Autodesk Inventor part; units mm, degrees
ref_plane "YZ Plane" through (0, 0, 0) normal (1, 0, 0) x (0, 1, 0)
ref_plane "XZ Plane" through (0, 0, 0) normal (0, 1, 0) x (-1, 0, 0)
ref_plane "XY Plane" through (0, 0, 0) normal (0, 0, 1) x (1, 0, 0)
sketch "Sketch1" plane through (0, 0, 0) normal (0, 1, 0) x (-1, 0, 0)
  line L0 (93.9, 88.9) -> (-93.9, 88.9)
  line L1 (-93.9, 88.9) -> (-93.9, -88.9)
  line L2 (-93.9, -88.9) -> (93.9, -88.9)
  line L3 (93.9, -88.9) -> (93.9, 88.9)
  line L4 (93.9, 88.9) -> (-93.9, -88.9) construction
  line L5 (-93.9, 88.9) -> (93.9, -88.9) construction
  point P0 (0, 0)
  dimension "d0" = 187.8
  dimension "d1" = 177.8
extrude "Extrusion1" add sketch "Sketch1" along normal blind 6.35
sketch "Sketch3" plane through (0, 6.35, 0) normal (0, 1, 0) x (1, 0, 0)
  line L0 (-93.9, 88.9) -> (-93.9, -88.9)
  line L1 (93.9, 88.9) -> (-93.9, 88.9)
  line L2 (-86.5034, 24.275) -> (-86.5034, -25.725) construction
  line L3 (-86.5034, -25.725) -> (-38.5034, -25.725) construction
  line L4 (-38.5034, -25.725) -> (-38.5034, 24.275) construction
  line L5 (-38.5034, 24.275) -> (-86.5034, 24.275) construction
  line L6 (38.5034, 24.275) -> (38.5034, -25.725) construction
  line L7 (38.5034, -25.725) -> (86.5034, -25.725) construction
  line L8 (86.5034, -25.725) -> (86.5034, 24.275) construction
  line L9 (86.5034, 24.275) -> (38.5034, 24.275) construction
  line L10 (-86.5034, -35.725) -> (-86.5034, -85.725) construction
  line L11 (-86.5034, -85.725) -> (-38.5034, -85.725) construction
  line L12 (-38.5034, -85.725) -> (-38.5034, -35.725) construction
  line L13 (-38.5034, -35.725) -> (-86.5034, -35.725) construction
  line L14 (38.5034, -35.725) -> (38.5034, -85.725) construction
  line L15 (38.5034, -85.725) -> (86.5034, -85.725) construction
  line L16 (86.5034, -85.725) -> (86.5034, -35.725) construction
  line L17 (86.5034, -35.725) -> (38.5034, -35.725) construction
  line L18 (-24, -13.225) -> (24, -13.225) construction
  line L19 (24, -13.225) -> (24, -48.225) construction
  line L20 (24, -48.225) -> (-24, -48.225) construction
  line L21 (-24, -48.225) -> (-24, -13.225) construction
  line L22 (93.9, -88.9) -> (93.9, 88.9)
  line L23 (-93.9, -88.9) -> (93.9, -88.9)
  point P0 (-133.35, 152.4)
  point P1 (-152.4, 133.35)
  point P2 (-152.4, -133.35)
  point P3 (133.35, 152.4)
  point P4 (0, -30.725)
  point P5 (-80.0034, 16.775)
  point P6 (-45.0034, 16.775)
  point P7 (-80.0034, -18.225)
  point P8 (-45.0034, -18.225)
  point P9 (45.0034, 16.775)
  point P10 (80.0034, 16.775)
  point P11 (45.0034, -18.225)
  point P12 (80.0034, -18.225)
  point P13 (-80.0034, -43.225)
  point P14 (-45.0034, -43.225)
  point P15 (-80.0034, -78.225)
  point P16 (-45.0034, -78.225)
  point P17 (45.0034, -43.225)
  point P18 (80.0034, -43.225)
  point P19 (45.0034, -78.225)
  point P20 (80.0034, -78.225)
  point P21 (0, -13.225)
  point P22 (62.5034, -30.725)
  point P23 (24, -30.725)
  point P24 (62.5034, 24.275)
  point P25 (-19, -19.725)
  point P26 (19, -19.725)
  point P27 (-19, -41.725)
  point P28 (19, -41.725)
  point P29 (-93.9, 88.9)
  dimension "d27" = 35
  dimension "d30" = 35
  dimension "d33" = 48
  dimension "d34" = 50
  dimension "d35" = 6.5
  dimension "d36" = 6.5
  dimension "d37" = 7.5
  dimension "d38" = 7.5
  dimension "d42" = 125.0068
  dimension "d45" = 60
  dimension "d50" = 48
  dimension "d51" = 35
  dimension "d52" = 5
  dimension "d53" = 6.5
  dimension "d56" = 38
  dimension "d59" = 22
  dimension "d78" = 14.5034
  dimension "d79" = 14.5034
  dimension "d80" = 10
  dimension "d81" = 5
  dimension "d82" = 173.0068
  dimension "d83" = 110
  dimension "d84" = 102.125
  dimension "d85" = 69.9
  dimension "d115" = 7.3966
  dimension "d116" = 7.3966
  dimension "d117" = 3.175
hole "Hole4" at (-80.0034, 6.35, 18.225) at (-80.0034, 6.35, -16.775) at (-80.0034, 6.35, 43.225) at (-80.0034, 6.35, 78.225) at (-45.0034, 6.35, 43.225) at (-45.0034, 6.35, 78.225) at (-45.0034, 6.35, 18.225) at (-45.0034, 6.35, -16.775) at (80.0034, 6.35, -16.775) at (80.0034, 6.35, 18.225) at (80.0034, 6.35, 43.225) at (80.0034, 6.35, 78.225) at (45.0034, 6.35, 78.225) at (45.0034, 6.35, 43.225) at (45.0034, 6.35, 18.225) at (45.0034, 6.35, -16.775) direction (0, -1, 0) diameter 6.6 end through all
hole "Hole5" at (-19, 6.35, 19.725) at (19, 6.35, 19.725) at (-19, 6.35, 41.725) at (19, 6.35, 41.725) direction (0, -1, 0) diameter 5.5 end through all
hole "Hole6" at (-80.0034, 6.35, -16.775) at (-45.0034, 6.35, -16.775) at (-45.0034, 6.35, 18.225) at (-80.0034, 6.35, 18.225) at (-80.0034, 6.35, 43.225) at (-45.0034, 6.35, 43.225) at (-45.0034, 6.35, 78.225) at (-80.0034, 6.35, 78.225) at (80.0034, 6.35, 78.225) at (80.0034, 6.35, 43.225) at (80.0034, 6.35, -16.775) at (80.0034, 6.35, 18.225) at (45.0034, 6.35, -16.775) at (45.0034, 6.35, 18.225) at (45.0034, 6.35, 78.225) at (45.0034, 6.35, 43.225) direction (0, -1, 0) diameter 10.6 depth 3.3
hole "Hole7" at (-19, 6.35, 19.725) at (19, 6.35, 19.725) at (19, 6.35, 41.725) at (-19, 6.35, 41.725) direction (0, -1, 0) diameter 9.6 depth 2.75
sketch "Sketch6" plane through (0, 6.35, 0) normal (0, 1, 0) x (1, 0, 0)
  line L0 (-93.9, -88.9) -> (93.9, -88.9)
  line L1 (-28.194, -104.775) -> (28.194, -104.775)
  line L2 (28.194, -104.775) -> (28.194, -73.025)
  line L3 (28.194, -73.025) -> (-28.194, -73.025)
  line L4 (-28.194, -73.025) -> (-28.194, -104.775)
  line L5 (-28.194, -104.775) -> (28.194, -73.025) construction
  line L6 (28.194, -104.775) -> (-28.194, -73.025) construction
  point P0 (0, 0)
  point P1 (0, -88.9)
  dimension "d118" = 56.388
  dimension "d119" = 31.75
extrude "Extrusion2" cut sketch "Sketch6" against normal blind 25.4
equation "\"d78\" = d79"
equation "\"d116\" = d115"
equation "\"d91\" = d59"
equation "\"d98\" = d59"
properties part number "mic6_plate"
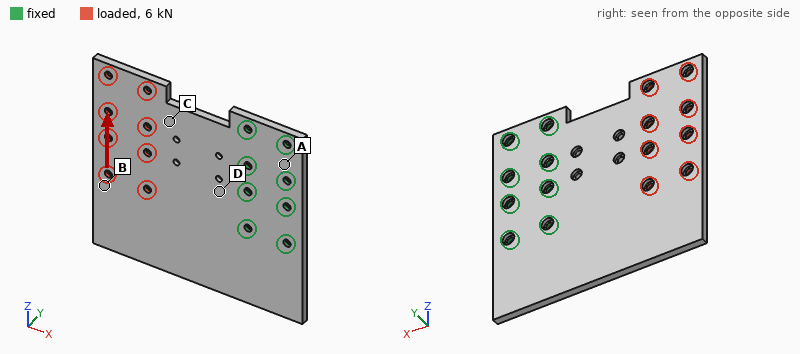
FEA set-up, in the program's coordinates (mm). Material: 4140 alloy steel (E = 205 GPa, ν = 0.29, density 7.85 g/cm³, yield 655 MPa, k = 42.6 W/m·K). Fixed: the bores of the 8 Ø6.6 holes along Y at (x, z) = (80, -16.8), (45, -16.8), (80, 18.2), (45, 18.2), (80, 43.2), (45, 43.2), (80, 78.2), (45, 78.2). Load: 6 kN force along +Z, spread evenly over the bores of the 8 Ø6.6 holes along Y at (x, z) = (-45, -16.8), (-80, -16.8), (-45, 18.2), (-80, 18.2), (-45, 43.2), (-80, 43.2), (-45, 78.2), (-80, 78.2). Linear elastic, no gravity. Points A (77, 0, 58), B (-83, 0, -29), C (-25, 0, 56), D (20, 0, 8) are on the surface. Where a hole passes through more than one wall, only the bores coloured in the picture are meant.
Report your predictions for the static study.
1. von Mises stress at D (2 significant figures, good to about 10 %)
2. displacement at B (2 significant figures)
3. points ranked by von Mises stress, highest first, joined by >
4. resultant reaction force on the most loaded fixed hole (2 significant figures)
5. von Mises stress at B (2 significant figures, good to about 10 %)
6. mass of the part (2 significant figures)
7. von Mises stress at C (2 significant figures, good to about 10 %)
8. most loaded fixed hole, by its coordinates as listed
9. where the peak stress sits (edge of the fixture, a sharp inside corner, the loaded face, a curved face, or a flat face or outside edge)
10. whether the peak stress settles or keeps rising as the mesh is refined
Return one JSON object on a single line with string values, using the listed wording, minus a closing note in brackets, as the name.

{"von Mises stress at D": "30 MPa", "displacement at B": "0.047 mm", "points ranked by von Mises stress, highest first, joined by >": "D > C > B > A", "resultant reaction force on the most loaded fixed hole": "5.8 kN", "von Mises stress at B": "12 MPa", "mass of the part": "1.6 kg", "von Mises stress at C": "22 MPa", "most loaded fixed hole, by its coordinates as listed": "(45, -16.8)", "where the peak stress sits": "edge of the fixture", "whether the peak stress settles or keeps rising as the mesh is refined": "keeps rising"}
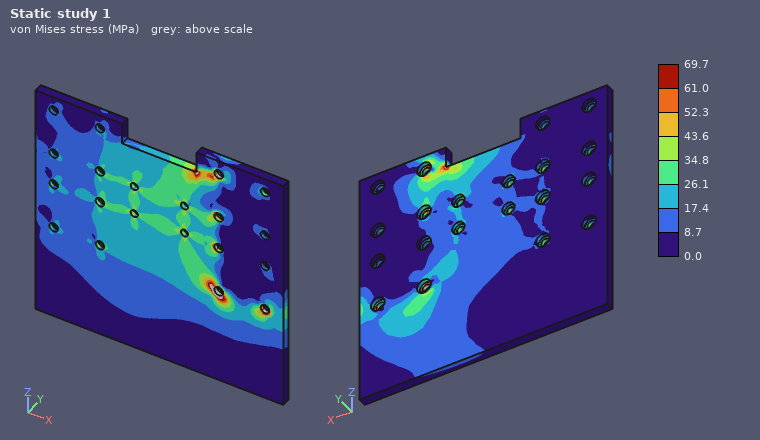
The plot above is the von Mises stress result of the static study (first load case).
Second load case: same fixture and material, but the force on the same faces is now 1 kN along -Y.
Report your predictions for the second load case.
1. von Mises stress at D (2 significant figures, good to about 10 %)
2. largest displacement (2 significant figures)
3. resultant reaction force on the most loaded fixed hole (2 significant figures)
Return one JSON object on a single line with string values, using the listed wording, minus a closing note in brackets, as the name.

{"von Mises stress at D": "86 MPa", "largest displacement": "1.2 mm", "resultant reaction force on the most loaded fixed hole": "2.0 kN"}
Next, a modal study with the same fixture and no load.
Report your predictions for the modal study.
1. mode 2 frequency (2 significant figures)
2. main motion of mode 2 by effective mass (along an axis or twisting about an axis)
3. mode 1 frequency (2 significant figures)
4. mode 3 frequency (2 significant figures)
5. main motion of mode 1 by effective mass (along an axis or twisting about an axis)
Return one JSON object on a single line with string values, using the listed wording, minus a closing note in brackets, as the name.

{"mode 2 frequency": "440 Hz", "main motion of mode 2 by effective mass": "twisting about X", "mode 1 frequency": "240 Hz", "mode 3 frequency": "940 Hz", "main motion of mode 1 by effective mass": "along Y"}
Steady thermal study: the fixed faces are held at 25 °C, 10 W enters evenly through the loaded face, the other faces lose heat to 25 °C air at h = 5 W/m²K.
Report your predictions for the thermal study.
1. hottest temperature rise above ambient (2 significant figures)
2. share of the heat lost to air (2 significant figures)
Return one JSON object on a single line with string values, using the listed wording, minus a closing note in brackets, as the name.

{"hottest temperature rise above ambient": "28 K", "share of the heat lost to air": "36 %"}
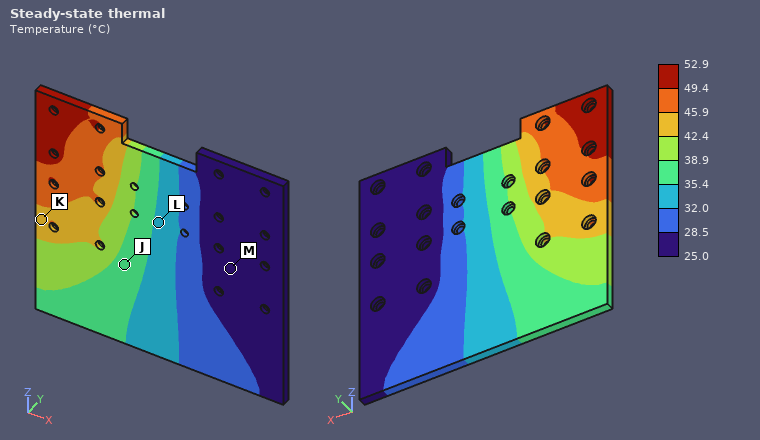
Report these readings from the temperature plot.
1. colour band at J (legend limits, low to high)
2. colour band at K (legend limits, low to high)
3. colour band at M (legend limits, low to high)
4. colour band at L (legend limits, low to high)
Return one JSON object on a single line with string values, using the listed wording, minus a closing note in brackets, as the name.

{"colour band at J": "35.4 to 38.9 °C", "colour band at K": "42.4 to 45.9 °C", "colour band at M": "25.0 to 28.5 °C", "colour band at L": "32.0 to 35.4 °C"}
